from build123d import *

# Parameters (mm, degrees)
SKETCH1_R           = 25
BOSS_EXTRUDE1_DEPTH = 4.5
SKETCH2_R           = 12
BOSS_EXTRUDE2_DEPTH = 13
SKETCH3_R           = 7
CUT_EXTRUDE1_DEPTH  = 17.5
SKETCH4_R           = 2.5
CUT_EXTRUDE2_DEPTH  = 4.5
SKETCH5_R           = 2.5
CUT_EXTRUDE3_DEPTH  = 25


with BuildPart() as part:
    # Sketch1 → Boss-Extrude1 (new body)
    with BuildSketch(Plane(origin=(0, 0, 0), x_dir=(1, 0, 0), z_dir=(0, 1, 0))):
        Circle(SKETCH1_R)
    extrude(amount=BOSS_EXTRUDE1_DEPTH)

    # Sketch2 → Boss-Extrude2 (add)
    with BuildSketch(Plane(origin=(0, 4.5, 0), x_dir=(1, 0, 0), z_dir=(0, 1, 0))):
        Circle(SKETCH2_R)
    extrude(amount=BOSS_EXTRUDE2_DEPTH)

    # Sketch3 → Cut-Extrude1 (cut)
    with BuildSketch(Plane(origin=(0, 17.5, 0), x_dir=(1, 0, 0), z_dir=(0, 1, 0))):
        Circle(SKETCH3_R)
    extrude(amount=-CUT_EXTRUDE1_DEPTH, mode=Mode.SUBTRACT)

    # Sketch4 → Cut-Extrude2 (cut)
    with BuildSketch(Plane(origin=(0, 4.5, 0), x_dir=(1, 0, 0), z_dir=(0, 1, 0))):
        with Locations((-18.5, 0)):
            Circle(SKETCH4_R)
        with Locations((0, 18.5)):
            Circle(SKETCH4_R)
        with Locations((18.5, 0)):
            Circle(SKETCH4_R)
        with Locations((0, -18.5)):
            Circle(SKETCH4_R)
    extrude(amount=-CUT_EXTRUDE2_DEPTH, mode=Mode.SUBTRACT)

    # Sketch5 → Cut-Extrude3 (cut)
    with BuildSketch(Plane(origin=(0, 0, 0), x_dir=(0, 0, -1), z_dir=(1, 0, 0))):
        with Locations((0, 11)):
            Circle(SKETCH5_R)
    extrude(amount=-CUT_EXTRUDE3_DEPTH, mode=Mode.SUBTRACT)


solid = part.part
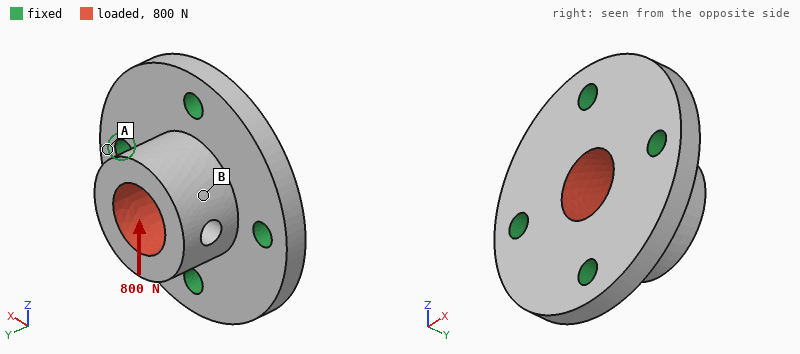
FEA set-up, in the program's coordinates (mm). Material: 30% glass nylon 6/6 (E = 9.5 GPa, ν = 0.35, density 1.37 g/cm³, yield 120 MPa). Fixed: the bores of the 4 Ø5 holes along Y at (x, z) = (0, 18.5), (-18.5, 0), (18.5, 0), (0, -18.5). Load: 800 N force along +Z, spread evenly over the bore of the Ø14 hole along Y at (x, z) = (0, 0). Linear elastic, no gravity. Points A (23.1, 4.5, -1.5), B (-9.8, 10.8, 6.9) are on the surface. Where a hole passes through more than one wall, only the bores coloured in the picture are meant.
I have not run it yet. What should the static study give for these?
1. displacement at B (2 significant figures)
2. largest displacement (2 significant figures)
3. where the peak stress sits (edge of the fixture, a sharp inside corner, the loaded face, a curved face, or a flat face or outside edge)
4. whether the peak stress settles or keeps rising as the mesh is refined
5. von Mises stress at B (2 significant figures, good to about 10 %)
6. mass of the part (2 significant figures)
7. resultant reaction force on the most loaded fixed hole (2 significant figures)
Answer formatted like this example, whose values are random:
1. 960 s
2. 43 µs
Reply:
1. 14 µm
2. 25 µm
3. edge of the fixture
4. keeps rising
5. 3.0 MPa
6. 16 g
7. 300 N
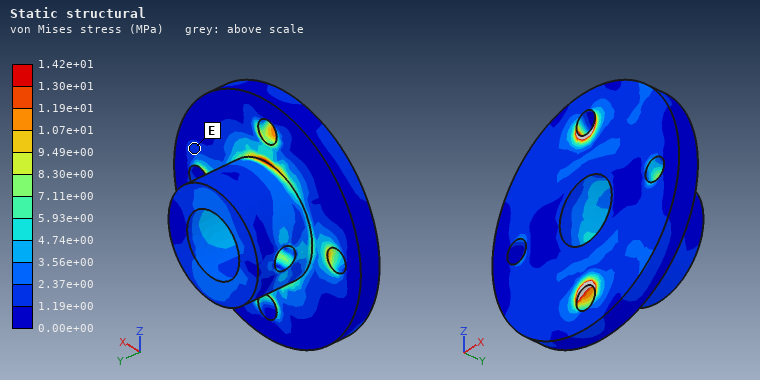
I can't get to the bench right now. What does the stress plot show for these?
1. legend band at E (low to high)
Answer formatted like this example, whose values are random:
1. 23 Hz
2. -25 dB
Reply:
1. 1.19e+00 to 2.37e+00 MPa
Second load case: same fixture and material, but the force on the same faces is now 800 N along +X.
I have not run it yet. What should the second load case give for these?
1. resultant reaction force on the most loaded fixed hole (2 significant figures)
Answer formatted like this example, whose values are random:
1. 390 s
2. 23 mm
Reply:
1. 300 N
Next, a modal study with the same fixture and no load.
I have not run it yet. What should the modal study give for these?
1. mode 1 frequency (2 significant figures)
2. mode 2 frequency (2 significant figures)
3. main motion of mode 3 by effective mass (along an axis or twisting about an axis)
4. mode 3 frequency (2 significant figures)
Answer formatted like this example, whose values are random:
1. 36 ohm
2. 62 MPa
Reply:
1. 11 kHz
2. 11 kHz
3. along Y
4. 12 kHz
